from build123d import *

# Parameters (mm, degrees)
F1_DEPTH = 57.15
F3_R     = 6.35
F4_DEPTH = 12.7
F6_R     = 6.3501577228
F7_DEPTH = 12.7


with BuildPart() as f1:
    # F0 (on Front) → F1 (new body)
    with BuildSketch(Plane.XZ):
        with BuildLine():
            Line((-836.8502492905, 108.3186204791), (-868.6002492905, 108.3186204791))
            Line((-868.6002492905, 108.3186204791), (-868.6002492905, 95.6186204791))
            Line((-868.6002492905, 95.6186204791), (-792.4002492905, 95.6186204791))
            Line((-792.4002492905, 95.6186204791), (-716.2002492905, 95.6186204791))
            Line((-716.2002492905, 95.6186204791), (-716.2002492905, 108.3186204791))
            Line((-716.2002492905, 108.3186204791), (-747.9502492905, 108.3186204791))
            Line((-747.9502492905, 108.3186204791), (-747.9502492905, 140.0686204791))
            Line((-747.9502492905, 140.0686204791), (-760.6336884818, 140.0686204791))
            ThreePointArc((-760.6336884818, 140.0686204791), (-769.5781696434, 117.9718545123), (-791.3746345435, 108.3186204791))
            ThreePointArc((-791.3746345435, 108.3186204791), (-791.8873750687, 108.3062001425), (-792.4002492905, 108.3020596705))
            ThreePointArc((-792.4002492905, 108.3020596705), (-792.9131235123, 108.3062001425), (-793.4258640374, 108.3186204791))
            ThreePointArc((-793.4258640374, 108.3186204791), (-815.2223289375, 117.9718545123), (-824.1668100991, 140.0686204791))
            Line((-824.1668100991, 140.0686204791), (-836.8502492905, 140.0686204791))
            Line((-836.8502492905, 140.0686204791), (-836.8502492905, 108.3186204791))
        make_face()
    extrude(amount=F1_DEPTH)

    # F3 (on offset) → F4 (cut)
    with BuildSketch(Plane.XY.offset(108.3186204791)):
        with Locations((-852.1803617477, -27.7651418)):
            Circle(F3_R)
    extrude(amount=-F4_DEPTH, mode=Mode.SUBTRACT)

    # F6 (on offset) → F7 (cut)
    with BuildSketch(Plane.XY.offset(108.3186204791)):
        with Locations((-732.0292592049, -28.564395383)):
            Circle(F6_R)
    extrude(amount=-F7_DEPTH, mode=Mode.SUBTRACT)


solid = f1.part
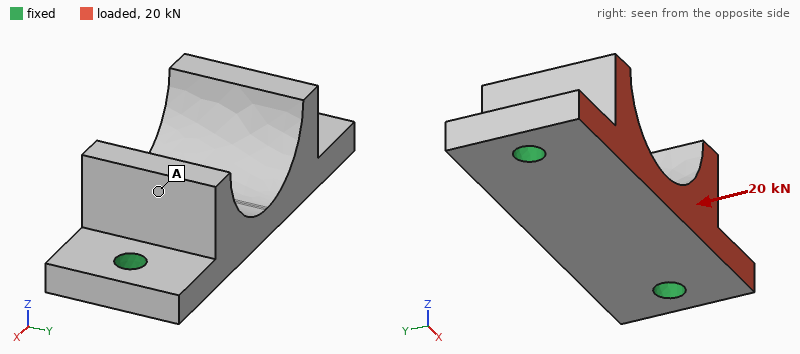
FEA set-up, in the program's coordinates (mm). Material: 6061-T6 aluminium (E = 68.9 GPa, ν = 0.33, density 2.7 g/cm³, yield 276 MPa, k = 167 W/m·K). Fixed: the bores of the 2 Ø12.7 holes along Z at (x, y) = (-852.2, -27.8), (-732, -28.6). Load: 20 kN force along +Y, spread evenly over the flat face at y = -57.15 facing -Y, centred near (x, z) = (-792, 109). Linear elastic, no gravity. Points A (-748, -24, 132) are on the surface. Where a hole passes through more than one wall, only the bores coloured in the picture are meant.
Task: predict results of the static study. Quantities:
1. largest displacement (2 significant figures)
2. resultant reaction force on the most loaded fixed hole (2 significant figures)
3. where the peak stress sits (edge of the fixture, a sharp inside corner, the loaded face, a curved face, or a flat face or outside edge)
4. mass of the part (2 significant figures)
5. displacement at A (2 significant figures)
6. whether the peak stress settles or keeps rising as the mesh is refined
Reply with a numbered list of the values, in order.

1. 79 µm
2. 10 kN
3. edge of the fixture
4. 480 g
5. 54 µm
6. keeps rising
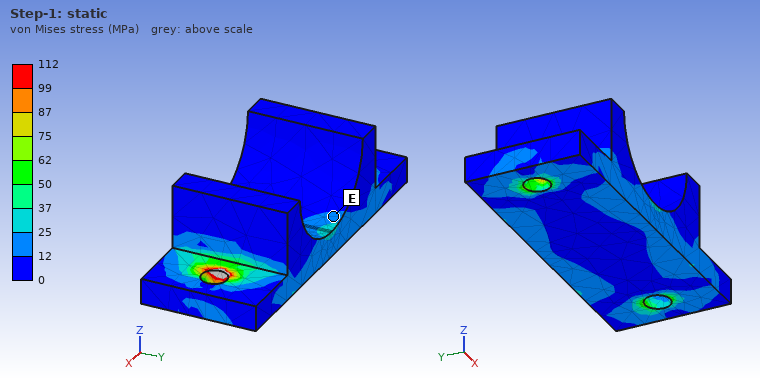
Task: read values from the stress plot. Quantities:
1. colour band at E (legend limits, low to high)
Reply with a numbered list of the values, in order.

1. 12 to 25 MPa
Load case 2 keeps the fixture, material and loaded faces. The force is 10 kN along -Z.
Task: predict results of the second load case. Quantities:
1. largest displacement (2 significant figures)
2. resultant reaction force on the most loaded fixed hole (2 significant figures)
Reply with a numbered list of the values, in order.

1. 0.13 mm
2. 5.2 kN
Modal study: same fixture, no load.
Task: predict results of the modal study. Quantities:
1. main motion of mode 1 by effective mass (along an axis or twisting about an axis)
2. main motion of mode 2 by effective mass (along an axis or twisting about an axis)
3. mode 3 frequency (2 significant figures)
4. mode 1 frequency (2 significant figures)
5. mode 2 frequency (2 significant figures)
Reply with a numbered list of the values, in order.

1. along Z
2. along Y
3. 6300 Hz
4. 3400 Hz
5. 3800 Hz
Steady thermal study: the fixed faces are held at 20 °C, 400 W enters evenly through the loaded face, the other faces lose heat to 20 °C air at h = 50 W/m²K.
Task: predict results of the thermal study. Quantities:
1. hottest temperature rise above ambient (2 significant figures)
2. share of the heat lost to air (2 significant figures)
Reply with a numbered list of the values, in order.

1. 53 K
2. 9.3 %
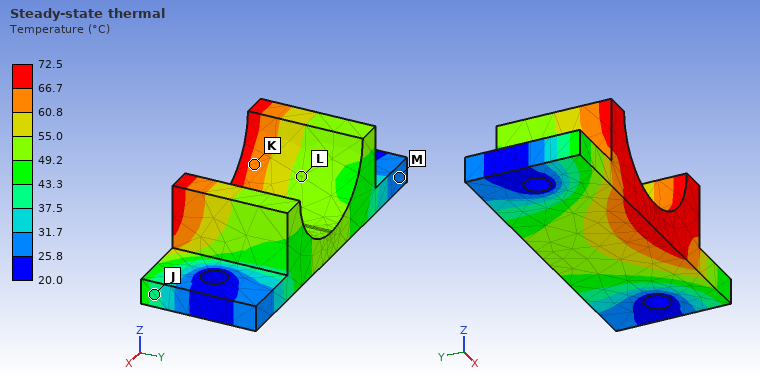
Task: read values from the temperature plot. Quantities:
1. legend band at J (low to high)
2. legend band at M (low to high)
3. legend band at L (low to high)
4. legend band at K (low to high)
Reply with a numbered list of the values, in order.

1. 37.5 to 43.3 °C
2. 25.8 to 31.7 °C
3. 49.2 to 55.0 °C
4. 60.8 to 66.7 °C
